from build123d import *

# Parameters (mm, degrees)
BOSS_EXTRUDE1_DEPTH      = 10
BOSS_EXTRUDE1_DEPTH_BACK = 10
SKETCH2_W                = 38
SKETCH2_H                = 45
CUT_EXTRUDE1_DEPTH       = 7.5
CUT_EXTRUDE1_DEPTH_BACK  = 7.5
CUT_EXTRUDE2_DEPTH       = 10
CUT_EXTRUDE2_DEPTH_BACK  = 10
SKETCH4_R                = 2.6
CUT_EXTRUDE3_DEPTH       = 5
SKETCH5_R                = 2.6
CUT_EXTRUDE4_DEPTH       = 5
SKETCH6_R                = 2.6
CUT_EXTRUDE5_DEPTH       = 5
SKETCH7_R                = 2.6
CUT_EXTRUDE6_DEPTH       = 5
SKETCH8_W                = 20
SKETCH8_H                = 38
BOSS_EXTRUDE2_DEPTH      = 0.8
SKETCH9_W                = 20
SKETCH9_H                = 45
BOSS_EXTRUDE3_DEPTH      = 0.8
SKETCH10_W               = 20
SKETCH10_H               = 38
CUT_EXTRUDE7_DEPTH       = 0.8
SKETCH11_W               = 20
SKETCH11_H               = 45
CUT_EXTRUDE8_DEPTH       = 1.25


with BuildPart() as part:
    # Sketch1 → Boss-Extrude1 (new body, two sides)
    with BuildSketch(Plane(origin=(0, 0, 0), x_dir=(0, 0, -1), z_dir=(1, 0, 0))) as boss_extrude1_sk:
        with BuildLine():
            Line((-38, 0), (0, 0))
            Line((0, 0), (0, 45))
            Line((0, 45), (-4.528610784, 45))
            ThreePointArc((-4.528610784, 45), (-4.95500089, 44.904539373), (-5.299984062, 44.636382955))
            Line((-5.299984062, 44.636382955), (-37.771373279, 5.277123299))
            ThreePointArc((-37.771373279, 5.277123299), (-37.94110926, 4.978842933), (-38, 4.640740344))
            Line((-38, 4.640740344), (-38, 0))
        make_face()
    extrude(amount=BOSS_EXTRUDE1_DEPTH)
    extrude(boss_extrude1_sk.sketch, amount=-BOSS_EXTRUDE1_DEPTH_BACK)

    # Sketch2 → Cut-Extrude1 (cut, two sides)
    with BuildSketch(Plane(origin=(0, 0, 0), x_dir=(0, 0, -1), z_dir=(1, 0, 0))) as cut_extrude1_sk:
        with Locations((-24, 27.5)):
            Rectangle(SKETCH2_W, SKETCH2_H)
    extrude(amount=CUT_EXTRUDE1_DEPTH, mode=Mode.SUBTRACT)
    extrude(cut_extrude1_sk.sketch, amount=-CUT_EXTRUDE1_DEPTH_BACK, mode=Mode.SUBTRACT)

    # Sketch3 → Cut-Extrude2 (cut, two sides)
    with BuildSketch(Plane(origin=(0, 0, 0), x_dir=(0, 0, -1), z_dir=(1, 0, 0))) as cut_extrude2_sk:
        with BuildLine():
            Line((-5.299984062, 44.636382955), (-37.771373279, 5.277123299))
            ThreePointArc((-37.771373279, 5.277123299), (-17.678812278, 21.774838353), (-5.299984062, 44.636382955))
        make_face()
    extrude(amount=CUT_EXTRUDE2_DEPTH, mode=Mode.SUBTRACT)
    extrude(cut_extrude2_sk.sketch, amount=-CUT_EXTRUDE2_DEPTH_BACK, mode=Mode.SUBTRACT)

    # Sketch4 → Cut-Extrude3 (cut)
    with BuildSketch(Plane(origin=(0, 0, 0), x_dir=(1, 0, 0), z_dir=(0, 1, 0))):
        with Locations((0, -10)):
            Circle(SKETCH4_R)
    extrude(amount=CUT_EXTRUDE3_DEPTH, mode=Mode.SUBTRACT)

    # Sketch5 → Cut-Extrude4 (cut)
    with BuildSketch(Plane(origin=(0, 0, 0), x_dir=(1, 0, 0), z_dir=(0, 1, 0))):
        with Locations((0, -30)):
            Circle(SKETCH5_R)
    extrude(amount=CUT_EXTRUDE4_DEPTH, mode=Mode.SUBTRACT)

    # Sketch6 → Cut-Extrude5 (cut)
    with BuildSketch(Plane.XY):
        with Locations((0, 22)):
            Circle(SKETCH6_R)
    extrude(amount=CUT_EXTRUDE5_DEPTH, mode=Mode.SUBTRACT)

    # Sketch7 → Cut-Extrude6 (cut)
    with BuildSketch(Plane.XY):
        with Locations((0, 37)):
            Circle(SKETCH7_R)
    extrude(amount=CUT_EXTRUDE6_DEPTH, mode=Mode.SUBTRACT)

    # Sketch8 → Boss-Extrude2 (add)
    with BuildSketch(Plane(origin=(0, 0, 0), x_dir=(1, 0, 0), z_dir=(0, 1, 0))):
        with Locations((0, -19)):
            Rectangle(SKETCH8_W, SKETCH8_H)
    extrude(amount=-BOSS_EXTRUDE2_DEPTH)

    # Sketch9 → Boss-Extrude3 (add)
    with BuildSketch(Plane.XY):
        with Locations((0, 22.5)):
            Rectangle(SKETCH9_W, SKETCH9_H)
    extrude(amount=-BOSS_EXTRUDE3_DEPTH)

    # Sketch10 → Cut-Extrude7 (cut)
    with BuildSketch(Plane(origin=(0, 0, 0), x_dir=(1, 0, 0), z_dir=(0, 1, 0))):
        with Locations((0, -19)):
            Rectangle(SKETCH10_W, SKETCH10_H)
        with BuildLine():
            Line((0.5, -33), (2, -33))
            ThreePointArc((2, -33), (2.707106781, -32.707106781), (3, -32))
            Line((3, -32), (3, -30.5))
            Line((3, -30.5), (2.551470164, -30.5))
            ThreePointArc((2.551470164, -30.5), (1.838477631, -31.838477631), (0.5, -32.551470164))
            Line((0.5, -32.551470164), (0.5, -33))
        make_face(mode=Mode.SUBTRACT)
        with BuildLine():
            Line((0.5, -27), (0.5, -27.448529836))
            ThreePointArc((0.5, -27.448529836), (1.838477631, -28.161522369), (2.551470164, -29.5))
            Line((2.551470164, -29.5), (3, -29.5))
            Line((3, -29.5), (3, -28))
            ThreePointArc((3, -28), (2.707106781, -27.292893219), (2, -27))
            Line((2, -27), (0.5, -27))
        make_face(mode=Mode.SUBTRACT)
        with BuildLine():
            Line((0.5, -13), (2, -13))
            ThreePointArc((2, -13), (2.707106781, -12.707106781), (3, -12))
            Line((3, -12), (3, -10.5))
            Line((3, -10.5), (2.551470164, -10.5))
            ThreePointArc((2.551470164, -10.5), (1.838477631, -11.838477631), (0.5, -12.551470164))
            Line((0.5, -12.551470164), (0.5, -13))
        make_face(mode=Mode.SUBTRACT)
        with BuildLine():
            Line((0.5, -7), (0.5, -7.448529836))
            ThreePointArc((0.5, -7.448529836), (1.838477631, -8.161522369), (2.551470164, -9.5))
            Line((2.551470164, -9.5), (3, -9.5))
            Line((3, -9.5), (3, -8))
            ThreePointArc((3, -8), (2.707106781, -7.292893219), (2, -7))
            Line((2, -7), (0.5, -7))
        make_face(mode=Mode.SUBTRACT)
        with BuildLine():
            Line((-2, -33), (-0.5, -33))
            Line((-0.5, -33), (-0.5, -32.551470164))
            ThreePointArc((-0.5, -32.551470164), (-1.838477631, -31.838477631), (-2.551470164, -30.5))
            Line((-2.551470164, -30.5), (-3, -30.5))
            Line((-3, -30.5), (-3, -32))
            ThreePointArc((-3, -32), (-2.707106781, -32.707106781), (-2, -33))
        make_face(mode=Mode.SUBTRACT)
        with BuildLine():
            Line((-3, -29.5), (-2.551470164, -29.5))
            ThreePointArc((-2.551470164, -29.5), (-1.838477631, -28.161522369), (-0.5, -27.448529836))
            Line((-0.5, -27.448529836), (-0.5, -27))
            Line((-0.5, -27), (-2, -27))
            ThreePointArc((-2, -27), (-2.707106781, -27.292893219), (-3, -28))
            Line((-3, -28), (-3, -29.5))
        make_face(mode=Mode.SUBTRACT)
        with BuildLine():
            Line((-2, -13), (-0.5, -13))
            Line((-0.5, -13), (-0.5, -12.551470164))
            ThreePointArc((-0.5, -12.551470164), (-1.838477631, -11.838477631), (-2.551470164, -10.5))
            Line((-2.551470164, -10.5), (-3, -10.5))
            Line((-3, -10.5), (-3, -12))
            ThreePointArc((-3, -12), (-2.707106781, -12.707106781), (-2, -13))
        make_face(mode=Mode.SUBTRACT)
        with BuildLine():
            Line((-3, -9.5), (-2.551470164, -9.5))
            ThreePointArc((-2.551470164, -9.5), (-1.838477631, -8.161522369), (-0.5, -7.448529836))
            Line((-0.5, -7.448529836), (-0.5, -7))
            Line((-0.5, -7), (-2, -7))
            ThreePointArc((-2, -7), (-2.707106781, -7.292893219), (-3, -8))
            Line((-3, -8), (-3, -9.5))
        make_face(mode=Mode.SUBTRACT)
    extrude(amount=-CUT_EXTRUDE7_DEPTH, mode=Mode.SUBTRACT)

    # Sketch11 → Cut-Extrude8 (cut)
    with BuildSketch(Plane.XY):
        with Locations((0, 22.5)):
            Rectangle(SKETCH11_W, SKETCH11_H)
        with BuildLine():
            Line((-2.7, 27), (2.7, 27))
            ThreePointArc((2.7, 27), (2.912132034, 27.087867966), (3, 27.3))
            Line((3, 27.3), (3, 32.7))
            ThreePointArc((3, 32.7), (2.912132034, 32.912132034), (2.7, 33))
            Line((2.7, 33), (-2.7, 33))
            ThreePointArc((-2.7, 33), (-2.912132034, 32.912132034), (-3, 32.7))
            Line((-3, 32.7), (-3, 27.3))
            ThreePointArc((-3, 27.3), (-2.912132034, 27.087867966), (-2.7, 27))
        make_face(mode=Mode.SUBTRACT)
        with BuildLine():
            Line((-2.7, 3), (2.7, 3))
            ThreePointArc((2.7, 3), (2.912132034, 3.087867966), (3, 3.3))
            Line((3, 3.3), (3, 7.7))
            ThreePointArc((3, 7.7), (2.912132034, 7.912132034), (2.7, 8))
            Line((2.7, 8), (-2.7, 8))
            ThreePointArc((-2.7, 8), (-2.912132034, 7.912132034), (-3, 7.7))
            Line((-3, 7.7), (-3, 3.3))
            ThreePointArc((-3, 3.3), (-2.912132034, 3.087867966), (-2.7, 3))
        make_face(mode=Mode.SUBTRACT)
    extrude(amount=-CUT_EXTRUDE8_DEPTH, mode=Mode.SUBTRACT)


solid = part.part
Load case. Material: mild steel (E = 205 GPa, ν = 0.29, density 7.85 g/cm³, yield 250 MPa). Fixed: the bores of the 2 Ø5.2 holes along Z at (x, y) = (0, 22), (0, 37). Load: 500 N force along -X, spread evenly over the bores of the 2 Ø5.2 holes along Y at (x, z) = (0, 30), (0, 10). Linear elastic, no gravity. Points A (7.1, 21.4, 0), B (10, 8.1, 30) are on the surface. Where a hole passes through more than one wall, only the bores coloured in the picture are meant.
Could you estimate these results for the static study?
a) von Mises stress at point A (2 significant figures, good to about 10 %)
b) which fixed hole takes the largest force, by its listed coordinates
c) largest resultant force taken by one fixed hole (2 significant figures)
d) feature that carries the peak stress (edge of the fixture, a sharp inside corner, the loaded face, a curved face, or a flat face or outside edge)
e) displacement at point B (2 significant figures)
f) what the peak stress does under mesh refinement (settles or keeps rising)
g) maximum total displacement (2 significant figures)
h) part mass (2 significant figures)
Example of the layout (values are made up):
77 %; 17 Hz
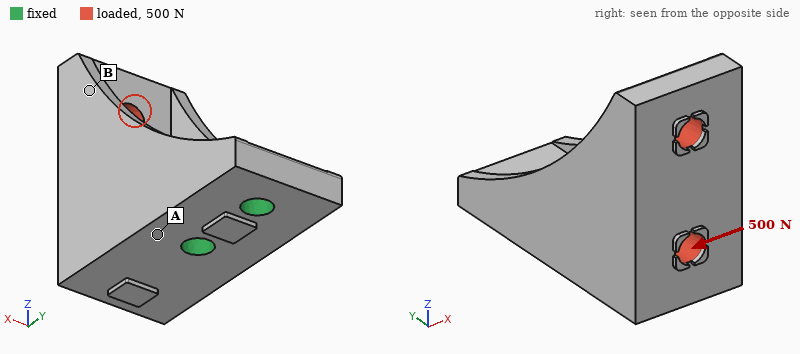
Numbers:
33 MPa; (0, 22); 870 N; edge of the fixture; 39 µm; keeps rising; 46 µm; 78 g
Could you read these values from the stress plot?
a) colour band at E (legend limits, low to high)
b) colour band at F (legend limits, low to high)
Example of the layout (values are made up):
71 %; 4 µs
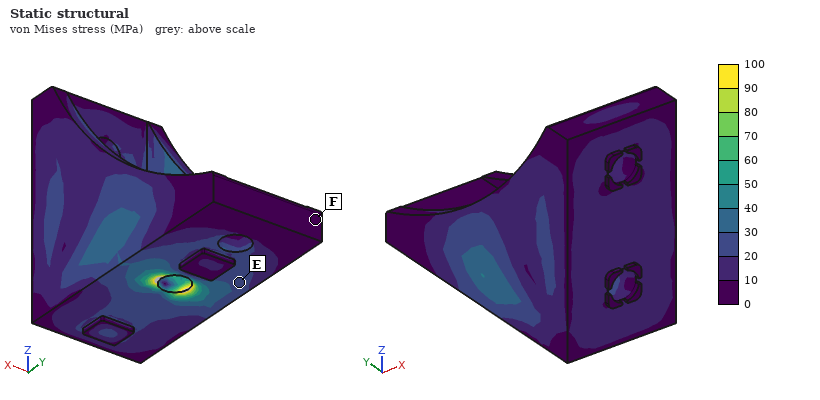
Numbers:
20 to 30 MPa; 0 to 10 MPa
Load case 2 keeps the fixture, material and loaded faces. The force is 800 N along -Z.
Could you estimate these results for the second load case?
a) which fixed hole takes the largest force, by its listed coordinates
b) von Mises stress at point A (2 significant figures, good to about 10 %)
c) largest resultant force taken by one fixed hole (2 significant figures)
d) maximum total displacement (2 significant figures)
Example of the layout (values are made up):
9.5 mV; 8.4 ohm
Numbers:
(0, 22); 30 MPa; 1.4 kN; 24 µm
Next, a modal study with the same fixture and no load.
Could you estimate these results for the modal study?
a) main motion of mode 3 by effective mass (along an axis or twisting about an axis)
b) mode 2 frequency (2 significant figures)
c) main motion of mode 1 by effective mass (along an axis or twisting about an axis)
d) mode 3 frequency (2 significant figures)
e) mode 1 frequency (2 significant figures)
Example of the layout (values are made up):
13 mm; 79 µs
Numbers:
along X; 4900 Hz; along X; 12 kHz; 3300 Hz
